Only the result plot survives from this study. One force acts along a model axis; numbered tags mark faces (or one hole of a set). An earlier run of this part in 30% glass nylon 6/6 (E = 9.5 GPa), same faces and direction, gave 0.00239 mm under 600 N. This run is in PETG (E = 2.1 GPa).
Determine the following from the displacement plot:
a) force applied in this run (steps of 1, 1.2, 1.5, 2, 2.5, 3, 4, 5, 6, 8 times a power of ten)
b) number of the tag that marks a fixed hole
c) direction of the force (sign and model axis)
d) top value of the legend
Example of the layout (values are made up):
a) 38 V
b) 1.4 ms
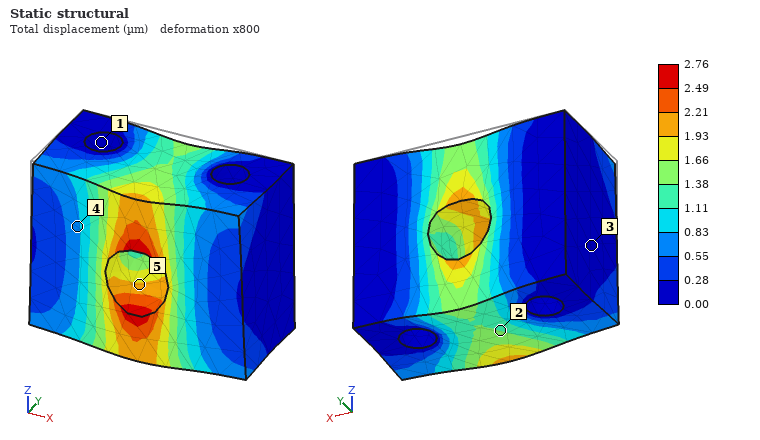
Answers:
a) 150 N
b) 1
c) -Z
d) 2.76 µm
